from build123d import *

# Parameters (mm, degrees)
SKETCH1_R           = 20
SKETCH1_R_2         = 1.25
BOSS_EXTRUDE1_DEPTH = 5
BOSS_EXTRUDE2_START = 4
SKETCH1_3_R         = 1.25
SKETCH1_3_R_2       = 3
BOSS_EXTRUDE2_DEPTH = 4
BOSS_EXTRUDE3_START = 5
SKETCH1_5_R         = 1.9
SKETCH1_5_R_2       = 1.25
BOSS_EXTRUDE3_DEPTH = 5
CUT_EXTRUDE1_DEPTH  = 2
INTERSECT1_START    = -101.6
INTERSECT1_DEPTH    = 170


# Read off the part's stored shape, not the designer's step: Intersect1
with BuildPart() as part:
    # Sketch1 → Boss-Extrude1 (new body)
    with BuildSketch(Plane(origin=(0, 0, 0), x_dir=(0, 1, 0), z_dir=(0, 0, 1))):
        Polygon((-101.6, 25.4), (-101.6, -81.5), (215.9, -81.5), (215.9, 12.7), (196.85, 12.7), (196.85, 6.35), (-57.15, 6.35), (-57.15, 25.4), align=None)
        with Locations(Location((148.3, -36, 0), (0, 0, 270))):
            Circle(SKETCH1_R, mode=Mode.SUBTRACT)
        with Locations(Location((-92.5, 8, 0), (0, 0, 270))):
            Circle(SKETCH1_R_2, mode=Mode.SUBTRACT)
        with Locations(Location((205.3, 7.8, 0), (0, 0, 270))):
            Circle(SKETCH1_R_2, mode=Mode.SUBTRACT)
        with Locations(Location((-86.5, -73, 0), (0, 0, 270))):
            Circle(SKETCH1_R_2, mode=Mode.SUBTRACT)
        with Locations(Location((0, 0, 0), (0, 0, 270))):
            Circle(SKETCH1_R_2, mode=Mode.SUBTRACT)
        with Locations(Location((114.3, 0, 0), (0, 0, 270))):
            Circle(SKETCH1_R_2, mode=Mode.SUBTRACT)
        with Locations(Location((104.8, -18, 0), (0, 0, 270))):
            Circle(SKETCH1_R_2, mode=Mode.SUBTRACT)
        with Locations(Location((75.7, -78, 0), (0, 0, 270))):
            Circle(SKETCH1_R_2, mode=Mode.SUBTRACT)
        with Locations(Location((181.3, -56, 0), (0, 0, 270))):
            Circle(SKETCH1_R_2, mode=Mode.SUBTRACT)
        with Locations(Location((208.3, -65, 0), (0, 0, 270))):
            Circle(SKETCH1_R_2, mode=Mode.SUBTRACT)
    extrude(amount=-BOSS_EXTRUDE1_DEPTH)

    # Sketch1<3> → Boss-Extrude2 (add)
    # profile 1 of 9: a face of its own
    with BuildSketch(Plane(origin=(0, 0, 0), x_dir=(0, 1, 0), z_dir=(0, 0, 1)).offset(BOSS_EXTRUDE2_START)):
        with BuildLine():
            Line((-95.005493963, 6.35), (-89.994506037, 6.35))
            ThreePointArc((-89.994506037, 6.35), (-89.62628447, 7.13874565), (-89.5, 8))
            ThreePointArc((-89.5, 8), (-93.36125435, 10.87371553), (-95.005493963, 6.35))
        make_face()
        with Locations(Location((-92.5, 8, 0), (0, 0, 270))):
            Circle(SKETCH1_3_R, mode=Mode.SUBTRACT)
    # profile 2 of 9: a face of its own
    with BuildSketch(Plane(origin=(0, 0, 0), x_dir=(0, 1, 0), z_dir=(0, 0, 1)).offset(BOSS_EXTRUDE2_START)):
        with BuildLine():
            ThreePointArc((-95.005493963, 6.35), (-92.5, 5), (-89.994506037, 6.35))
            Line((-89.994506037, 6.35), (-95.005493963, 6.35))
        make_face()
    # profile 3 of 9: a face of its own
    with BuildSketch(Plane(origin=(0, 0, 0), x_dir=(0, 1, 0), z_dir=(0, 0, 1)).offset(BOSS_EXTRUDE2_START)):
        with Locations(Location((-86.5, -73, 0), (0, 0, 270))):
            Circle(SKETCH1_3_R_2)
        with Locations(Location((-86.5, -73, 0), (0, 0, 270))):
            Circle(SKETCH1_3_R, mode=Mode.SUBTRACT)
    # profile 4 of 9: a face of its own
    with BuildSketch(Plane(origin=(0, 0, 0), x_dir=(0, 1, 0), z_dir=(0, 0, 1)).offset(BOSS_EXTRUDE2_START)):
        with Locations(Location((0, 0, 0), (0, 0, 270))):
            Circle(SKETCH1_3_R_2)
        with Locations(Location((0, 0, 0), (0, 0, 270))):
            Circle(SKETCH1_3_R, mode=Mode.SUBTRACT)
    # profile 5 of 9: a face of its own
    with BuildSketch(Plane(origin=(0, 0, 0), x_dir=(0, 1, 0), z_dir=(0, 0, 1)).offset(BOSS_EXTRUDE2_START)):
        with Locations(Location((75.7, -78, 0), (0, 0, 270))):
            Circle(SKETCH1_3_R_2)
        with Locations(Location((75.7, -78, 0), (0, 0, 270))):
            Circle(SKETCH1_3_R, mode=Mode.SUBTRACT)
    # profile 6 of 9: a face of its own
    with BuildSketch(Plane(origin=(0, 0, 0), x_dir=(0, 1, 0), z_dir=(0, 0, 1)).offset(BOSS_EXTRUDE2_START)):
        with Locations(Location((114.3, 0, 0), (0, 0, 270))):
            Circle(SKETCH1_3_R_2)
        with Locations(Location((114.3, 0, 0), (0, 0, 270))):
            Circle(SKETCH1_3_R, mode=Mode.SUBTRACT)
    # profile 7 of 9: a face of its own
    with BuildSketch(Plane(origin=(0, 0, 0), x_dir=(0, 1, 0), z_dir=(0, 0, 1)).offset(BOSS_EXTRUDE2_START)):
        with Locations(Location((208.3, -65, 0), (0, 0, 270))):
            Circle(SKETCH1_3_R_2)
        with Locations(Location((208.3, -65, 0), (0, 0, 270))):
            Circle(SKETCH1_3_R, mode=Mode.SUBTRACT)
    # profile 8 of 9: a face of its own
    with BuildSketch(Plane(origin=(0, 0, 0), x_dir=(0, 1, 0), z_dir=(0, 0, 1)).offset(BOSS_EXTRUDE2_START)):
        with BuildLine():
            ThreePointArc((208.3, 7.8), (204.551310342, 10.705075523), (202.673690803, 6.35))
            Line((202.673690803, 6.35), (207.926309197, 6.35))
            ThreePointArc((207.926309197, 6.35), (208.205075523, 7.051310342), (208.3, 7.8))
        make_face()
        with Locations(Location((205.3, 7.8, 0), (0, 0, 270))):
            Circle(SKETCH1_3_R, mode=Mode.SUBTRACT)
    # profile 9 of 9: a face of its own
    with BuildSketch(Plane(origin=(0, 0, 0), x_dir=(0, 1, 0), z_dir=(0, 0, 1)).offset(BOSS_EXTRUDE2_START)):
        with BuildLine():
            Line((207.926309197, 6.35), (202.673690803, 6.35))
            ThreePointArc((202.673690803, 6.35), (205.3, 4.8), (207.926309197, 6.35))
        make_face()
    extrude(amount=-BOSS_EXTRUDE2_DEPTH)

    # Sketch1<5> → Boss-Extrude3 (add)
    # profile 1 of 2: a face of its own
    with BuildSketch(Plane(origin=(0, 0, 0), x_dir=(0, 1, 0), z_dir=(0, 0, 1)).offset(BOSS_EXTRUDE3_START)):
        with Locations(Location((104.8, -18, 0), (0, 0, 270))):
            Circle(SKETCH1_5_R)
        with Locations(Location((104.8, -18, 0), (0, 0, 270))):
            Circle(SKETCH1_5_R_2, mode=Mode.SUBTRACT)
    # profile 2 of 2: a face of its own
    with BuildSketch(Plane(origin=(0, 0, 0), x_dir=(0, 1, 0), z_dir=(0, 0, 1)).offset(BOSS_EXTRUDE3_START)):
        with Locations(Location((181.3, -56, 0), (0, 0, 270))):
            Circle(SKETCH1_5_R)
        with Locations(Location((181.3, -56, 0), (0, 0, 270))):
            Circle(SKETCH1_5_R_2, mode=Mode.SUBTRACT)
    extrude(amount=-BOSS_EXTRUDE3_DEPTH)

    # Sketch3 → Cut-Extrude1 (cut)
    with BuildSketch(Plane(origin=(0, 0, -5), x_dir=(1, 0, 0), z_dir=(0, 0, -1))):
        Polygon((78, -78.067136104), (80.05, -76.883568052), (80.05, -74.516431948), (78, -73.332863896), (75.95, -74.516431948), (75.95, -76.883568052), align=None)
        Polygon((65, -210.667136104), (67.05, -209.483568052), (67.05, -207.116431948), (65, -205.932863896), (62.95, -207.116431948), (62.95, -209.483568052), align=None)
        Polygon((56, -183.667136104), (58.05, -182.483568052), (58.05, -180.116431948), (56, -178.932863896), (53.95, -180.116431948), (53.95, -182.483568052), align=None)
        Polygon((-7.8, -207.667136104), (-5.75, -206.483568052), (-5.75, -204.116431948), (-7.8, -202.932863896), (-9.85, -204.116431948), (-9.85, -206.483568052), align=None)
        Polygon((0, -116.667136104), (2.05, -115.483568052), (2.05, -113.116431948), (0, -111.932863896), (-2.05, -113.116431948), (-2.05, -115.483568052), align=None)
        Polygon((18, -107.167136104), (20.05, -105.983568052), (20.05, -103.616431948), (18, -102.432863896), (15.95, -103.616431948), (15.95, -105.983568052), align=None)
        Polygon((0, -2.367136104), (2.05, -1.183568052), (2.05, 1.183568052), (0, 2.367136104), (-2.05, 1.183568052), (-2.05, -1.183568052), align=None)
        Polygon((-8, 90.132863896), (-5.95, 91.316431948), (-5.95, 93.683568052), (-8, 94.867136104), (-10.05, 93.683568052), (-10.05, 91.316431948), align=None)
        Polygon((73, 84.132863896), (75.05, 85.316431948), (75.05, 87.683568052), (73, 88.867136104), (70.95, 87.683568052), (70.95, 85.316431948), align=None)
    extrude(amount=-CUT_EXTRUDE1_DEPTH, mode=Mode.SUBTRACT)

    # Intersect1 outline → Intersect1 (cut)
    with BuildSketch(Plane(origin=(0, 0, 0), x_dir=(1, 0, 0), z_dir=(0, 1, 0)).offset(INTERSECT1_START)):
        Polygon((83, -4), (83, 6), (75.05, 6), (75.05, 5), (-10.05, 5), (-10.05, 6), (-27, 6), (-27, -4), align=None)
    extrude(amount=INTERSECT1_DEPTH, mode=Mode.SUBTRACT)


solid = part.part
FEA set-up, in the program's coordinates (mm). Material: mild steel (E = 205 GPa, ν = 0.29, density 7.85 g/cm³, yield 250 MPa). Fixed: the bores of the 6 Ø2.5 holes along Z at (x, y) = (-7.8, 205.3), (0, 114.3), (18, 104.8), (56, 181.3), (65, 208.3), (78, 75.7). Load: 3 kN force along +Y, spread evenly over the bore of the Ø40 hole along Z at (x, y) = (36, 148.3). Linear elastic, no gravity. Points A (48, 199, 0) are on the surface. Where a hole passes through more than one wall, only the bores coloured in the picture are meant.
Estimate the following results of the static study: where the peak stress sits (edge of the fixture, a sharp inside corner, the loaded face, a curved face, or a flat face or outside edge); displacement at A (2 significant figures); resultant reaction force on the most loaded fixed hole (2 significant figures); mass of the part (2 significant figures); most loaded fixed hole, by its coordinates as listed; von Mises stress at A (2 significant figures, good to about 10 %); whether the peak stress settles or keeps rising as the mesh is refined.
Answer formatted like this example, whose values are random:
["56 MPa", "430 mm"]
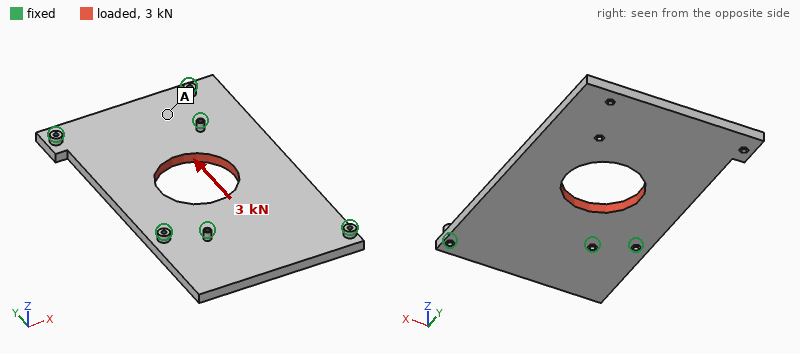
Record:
["edge of the fixture", "0.64 µm", "790 N", "470 g", "(56, 181.3)", "3.2 MPa", "keeps rising"]
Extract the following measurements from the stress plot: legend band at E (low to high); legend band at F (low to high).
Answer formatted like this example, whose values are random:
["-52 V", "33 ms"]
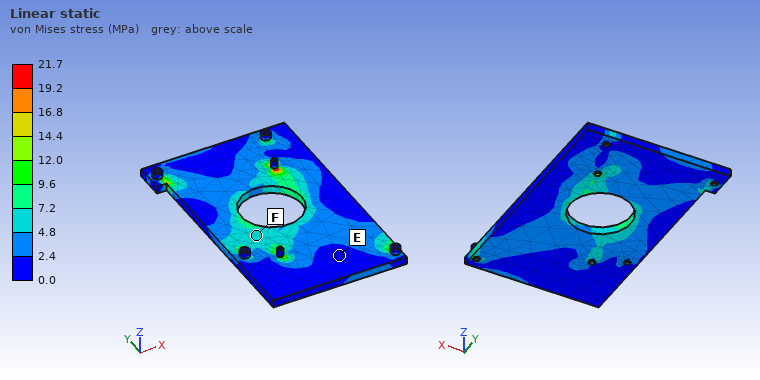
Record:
["0.0 to 2.4 MPa", "4.8 to 7.2 MPa"]
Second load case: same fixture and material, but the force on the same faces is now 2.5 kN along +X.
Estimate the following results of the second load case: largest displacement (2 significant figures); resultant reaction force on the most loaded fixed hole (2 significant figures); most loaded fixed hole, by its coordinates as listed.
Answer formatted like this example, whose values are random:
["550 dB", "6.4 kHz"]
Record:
["2.3 µm", "840 N", "(56, 181.3)"]
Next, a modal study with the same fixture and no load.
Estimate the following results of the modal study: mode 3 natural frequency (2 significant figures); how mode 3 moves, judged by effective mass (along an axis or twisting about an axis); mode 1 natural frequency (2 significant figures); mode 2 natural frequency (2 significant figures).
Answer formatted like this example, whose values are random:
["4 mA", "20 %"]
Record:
["3000 Hz", "along Z", "2000 Hz", "2700 Hz"]
